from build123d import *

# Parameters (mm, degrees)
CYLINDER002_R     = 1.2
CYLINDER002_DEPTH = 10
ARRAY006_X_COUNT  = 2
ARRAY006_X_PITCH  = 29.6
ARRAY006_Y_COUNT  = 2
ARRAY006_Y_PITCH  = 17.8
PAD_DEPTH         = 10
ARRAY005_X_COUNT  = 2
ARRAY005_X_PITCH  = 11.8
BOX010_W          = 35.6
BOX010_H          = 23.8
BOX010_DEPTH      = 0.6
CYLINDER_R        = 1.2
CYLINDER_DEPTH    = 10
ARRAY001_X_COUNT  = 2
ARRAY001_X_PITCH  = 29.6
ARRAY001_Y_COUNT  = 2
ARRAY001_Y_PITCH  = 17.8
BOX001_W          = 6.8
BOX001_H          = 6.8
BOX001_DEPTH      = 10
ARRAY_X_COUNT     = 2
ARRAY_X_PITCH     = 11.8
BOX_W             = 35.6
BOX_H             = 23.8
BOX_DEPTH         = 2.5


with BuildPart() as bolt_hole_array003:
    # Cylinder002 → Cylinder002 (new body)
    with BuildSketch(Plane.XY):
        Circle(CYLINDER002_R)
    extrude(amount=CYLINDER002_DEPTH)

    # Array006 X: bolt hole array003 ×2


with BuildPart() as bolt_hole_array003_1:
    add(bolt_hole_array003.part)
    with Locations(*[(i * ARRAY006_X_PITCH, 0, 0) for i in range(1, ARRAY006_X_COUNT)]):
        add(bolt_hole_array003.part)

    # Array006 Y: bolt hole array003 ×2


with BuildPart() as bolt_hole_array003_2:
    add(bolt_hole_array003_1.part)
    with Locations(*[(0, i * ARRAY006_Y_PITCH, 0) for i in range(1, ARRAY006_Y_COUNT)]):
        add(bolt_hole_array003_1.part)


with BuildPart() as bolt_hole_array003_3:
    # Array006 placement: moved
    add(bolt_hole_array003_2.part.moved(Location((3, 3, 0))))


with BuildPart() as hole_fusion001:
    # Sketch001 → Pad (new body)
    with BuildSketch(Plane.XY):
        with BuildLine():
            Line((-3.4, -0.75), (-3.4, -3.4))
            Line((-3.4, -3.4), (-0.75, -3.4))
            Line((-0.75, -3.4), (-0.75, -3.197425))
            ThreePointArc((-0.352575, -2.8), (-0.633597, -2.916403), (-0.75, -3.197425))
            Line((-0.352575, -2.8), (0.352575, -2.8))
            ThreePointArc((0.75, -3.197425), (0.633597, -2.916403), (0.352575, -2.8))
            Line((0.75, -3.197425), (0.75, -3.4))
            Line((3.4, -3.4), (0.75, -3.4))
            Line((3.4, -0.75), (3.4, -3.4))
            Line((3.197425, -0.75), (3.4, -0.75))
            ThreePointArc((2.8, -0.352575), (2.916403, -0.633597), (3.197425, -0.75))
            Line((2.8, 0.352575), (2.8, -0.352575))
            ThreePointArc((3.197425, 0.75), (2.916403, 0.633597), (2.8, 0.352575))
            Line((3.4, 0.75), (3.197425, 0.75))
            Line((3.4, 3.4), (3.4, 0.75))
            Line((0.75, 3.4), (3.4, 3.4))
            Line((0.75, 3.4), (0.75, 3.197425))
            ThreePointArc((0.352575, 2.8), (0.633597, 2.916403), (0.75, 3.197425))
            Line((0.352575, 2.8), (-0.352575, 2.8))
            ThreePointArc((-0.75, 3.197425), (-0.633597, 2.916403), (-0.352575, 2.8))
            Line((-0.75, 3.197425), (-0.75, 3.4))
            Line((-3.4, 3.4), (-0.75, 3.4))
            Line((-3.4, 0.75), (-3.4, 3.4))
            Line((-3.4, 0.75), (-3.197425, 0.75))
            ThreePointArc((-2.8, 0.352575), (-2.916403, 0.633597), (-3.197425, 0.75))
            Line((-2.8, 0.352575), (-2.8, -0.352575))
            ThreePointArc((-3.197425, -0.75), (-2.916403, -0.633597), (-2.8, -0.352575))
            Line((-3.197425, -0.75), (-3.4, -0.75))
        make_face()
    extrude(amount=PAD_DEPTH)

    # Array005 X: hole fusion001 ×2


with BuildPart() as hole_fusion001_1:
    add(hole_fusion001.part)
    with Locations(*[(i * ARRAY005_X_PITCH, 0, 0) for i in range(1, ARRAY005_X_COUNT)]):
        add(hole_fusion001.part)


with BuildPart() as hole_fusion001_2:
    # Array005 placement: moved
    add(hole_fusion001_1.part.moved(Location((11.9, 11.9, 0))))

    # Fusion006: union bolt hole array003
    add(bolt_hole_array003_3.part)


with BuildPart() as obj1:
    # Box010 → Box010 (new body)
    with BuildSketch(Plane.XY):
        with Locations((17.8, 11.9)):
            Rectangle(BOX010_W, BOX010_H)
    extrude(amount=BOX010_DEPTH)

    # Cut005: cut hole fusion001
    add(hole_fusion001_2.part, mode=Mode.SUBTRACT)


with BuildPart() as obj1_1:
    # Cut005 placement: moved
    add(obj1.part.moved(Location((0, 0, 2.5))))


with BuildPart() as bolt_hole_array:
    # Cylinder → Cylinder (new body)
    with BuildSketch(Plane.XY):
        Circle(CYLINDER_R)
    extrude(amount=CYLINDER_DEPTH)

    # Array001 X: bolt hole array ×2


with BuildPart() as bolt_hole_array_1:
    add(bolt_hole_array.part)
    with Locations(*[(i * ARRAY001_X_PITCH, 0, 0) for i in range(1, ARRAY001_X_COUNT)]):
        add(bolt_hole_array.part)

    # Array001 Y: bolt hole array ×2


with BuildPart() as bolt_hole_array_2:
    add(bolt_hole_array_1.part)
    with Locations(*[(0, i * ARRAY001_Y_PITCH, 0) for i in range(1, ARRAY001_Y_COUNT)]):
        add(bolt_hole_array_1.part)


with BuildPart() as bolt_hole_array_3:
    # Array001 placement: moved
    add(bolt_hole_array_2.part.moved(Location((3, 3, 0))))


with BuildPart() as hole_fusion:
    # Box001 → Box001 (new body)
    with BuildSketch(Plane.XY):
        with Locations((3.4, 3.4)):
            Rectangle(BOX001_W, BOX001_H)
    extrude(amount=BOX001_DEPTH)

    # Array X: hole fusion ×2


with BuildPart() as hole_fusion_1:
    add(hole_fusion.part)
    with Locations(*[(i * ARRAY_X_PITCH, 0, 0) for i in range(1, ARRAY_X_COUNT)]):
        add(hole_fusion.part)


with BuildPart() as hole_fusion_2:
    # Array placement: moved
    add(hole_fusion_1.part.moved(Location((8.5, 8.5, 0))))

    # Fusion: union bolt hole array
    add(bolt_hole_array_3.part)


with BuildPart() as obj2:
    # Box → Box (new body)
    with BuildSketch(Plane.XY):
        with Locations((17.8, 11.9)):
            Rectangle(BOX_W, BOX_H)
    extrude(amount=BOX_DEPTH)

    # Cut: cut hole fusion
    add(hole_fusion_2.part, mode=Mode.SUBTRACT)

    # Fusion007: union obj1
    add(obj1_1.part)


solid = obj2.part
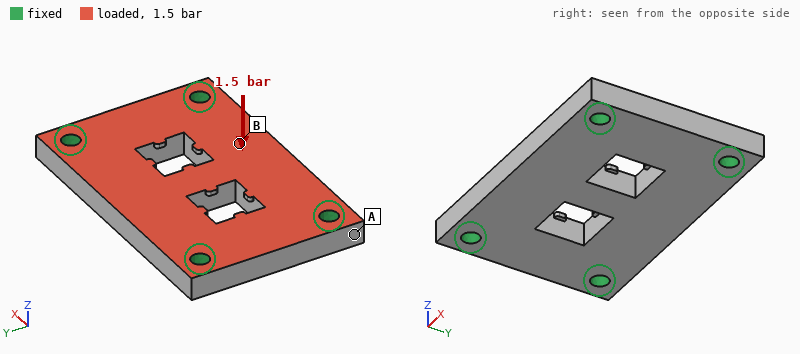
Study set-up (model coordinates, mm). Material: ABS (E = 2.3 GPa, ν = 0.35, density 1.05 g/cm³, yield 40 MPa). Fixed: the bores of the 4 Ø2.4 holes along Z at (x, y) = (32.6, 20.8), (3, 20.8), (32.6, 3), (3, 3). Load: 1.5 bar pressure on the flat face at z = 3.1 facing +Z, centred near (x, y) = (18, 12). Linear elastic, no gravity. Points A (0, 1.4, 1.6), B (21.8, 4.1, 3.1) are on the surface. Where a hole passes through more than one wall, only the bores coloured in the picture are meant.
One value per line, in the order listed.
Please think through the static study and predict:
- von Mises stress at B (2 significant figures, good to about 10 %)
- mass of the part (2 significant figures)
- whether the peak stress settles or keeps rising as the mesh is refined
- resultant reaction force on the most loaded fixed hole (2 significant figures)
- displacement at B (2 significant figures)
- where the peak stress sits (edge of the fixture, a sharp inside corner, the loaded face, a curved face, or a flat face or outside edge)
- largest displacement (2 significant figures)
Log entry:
2.8 MPa
2.4 g
keeps rising
28 N
56 µm
edge of the fixture
76 µm
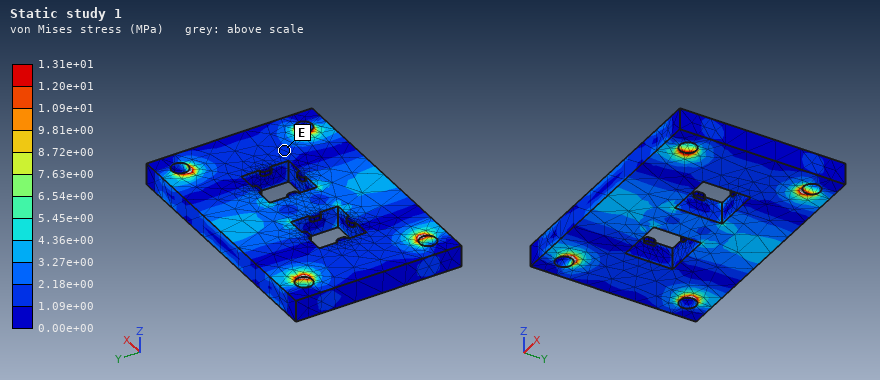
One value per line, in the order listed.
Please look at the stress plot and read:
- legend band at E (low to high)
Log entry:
1.09e+00 to 2.18e+00 MPa
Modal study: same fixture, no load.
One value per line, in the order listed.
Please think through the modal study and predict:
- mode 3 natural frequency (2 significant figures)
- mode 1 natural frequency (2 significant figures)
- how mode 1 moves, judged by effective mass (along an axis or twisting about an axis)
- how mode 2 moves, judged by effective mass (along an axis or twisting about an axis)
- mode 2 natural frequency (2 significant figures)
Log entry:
10 kHz
4700 Hz
along Z
twisting about X
6300 Hz
